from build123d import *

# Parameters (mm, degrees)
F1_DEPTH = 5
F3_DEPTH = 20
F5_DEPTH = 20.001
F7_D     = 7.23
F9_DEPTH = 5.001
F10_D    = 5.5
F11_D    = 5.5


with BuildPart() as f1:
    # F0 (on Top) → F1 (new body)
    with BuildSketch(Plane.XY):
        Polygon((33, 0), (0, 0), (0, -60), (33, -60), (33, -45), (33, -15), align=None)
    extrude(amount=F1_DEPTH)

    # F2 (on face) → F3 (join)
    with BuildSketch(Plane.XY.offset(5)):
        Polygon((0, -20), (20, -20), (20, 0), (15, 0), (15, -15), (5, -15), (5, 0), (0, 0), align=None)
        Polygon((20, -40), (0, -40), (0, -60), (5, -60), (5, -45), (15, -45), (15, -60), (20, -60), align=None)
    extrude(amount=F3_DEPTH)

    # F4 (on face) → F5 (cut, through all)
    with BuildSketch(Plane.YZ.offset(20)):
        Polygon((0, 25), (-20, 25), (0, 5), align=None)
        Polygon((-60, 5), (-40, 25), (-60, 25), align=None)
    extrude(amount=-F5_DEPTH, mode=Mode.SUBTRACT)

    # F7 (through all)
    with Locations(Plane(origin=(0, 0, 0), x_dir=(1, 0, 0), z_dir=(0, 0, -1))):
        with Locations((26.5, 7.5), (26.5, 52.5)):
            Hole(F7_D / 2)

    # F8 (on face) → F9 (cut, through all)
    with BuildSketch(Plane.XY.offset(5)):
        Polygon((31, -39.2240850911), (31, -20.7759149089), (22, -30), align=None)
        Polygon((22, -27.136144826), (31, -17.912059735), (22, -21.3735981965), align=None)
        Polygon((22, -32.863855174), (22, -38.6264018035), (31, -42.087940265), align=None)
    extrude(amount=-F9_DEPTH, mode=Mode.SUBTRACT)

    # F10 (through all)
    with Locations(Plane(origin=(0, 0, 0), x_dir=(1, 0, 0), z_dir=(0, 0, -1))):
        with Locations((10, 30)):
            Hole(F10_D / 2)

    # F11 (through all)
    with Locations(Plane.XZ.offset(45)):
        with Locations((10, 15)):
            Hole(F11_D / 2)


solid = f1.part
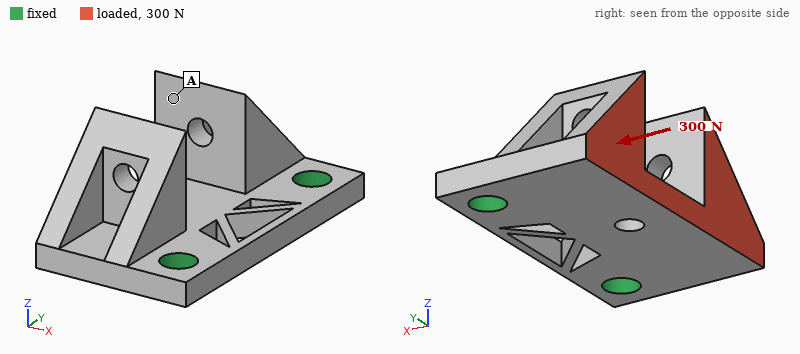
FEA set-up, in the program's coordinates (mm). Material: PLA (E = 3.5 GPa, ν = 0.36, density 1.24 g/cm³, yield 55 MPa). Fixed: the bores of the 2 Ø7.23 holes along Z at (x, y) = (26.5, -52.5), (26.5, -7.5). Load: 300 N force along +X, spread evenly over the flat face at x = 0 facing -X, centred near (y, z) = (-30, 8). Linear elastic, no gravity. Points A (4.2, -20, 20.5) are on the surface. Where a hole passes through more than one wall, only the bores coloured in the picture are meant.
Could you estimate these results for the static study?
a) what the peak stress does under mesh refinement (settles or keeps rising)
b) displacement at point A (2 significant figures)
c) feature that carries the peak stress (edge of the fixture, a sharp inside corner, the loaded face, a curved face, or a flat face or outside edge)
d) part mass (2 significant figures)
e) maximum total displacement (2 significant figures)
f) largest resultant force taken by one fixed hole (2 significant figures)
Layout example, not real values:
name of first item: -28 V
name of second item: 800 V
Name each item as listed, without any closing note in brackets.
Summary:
what the peak stress does under mesh refinement: keeps rising
displacement at point A: 0.22 mm
feature that carries the peak stress: edge of the fixture
part mass: 18 g
maximum total displacement: 0.27 mm
largest resultant force taken by one fixed hole: 160 N
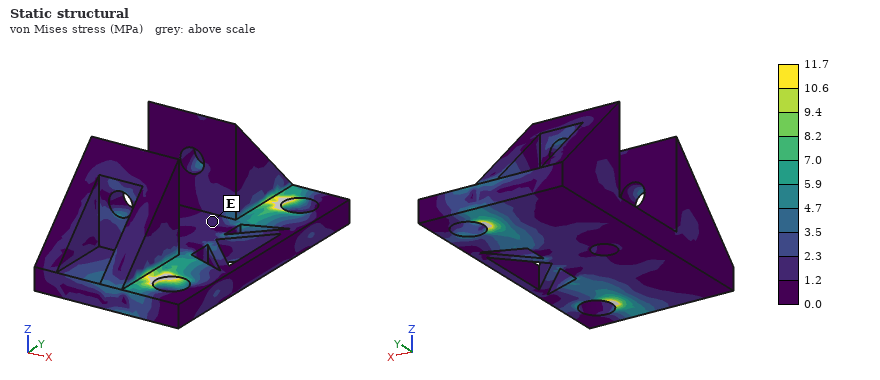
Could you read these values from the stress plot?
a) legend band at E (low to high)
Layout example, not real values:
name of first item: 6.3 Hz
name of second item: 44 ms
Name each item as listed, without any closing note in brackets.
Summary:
legend band at E: 1.2 to 2.3 MPa
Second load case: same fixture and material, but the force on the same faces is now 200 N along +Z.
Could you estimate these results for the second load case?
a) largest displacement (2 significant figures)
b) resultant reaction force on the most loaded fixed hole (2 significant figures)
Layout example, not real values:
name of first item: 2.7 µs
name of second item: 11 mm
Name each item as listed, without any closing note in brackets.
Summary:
largest displacement: 0.73 mm
resultant reaction force on the most loaded fixed hole: 100 N
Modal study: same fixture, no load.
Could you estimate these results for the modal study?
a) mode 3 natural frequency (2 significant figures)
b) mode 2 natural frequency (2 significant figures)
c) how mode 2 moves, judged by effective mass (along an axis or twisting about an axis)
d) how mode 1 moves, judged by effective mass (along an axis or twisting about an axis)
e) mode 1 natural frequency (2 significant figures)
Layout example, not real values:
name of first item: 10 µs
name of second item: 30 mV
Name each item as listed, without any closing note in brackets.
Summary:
mode 3 natural frequency: 2800 Hz
mode 2 natural frequency: 2000 Hz
how mode 2 moves, judged by effective mass: twisting about X
how mode 1 moves, judged by effective mass: along Z
mode 1 natural frequency: 1200 Hz
